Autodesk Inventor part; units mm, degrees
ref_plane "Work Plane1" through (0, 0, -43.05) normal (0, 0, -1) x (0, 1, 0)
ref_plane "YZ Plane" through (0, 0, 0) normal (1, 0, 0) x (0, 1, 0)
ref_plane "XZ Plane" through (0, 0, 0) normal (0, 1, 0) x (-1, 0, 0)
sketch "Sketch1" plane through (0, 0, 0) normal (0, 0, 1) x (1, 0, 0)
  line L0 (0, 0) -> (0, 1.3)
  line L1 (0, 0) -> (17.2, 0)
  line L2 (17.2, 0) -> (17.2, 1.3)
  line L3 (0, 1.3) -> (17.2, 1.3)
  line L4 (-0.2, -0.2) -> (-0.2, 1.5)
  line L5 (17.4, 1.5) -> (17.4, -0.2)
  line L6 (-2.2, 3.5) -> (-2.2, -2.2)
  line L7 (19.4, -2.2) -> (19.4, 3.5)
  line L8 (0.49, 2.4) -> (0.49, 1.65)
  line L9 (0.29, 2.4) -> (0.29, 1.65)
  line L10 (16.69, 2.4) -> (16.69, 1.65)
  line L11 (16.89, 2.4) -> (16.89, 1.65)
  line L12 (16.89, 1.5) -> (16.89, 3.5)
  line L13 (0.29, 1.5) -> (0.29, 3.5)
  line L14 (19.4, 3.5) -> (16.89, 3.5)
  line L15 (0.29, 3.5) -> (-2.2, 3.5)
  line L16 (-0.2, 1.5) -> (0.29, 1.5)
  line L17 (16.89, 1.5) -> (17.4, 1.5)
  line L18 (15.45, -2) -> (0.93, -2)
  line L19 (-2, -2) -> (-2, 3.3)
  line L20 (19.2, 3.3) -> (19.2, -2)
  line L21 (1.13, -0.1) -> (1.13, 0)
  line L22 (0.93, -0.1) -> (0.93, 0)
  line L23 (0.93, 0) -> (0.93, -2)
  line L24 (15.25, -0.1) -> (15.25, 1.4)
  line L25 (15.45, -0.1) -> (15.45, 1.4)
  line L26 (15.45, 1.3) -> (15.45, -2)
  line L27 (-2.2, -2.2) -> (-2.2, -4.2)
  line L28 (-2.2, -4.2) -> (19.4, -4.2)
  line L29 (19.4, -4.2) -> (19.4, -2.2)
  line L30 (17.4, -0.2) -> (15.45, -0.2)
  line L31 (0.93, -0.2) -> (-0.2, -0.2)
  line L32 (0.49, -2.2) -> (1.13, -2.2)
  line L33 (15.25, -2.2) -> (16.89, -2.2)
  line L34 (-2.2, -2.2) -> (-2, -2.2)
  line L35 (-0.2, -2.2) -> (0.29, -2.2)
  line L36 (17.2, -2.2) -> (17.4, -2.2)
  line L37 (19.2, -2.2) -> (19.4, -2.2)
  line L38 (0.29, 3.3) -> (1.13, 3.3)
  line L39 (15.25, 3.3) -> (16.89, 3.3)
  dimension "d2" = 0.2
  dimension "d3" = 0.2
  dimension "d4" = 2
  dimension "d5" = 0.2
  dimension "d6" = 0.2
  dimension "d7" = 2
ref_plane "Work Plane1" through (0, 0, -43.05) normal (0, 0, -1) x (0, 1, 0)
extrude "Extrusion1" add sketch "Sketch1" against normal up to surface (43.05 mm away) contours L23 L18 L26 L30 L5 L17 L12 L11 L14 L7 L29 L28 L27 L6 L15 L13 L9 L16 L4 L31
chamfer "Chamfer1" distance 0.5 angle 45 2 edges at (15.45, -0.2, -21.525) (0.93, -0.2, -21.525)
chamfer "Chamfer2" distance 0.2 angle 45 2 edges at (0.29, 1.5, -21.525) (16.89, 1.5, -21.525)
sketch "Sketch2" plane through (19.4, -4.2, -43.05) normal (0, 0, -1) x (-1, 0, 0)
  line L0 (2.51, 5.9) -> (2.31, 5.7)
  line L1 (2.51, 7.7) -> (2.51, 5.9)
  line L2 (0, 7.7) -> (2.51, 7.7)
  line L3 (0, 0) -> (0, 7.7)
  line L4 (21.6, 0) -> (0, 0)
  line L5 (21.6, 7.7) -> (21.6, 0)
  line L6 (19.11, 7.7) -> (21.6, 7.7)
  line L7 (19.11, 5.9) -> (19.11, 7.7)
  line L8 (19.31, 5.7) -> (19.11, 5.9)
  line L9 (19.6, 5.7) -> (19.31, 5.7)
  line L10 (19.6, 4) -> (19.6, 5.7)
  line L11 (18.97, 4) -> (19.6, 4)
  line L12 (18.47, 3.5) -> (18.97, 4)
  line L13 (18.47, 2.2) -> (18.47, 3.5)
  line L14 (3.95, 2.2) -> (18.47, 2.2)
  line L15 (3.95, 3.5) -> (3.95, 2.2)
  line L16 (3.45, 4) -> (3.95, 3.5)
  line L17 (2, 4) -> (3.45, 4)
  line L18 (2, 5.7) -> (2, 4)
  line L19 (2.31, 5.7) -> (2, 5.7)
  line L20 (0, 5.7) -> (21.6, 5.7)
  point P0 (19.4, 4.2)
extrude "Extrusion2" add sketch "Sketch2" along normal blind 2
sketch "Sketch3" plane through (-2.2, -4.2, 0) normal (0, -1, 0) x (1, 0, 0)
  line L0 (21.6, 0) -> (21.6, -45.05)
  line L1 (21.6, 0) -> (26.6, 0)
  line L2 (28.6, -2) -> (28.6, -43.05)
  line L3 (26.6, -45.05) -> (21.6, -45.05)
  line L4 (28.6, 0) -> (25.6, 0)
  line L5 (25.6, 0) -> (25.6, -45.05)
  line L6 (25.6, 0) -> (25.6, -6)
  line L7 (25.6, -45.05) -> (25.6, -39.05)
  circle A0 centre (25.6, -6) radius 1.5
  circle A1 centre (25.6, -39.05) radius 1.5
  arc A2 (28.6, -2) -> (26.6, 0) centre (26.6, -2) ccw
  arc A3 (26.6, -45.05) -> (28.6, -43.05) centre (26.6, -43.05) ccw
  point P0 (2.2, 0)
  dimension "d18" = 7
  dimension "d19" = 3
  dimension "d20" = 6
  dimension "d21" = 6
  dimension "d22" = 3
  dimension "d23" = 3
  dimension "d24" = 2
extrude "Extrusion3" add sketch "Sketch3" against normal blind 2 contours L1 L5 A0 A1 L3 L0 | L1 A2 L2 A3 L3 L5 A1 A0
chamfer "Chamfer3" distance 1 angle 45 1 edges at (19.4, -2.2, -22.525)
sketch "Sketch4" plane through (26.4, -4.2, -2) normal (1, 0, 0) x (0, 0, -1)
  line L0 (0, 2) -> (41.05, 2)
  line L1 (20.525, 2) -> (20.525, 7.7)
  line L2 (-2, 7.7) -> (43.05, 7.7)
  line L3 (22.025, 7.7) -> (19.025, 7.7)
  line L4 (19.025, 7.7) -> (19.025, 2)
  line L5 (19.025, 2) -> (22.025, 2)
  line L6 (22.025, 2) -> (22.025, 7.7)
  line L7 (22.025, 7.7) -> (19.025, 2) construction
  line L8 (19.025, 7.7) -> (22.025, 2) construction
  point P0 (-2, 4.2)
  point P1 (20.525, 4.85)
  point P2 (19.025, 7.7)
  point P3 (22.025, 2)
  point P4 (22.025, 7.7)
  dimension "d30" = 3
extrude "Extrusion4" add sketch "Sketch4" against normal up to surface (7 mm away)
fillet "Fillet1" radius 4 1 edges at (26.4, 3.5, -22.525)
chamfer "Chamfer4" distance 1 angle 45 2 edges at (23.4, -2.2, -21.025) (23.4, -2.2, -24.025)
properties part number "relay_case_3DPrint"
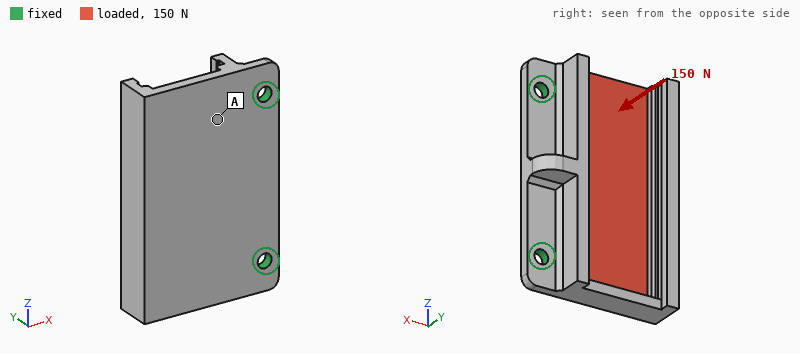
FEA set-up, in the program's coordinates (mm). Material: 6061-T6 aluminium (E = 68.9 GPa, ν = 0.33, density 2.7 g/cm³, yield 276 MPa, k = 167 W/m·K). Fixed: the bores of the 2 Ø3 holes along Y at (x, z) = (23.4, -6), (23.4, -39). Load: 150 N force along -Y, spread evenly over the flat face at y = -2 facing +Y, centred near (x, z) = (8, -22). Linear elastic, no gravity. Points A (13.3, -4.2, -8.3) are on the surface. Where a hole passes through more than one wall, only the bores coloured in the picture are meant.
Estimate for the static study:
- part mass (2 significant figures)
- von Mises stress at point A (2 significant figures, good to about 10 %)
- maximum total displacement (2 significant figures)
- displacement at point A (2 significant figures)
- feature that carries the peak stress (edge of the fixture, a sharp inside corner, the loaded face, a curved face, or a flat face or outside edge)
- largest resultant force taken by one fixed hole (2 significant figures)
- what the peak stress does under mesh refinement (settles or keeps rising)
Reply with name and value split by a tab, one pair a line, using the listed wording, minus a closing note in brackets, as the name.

part mass	12 g
von Mises stress at point A	21 MPa
maximum total displacement	0.17 mm
displacement at point A	0.048 mm
feature that carries the peak stress	edge of the fixture
largest resultant force taken by one fixed hole	85 N
what the peak stress does under mesh refinement	keeps rising
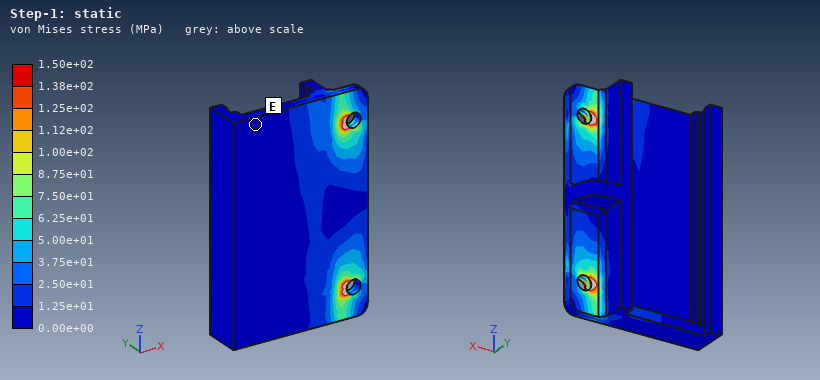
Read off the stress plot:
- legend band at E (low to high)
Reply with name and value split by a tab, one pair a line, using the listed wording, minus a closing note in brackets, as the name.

legend band at E	0.00e+00 to 1.25e+01 MPa
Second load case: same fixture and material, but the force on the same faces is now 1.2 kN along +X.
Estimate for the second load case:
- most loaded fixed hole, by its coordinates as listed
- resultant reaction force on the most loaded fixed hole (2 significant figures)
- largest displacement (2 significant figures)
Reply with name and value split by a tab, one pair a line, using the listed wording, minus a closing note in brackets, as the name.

most loaded fixed hole, by its coordinates as listed	(23.4, -6)
resultant reaction force on the most loaded fixed hole	650 N
largest displacement	0.14 mm
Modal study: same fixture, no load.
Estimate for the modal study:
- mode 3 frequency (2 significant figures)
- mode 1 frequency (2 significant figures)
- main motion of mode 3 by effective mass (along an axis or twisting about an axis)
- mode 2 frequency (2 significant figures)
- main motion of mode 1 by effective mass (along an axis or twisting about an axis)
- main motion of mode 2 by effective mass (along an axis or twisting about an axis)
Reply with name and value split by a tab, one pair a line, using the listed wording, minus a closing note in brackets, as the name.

mode 3 frequency	11 kHz
mode 1 frequency	1800 Hz
main motion of mode 3 by effective mass	along Y
mode 2 frequency	4100 Hz
main motion of mode 1 by effective mass	along Y
main motion of mode 2 by effective mass	twisting about X
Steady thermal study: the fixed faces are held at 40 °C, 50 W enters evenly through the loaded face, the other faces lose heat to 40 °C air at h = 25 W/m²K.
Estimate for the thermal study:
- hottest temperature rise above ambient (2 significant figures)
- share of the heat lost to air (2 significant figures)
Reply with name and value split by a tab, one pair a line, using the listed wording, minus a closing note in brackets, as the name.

hottest temperature rise above ambient	55 K
share of the heat lost to air	6.6 %
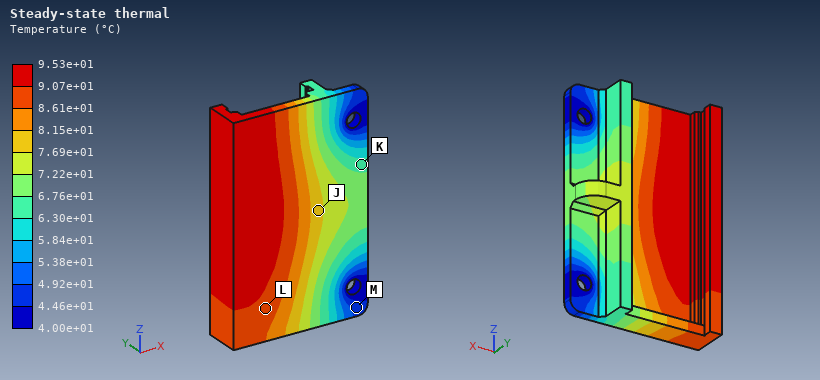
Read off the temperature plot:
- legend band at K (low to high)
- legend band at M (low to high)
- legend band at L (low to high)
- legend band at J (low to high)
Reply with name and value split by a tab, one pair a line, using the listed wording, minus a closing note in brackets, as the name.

legend band at K	6.30e+01 to 6.76e+01 °C
legend band at M	4.46e+01 to 4.92e+01 °C
legend band at L	8.61e+01 to 9.07e+01 °C
legend band at J	7.69e+01 to 8.15e+01 °C
